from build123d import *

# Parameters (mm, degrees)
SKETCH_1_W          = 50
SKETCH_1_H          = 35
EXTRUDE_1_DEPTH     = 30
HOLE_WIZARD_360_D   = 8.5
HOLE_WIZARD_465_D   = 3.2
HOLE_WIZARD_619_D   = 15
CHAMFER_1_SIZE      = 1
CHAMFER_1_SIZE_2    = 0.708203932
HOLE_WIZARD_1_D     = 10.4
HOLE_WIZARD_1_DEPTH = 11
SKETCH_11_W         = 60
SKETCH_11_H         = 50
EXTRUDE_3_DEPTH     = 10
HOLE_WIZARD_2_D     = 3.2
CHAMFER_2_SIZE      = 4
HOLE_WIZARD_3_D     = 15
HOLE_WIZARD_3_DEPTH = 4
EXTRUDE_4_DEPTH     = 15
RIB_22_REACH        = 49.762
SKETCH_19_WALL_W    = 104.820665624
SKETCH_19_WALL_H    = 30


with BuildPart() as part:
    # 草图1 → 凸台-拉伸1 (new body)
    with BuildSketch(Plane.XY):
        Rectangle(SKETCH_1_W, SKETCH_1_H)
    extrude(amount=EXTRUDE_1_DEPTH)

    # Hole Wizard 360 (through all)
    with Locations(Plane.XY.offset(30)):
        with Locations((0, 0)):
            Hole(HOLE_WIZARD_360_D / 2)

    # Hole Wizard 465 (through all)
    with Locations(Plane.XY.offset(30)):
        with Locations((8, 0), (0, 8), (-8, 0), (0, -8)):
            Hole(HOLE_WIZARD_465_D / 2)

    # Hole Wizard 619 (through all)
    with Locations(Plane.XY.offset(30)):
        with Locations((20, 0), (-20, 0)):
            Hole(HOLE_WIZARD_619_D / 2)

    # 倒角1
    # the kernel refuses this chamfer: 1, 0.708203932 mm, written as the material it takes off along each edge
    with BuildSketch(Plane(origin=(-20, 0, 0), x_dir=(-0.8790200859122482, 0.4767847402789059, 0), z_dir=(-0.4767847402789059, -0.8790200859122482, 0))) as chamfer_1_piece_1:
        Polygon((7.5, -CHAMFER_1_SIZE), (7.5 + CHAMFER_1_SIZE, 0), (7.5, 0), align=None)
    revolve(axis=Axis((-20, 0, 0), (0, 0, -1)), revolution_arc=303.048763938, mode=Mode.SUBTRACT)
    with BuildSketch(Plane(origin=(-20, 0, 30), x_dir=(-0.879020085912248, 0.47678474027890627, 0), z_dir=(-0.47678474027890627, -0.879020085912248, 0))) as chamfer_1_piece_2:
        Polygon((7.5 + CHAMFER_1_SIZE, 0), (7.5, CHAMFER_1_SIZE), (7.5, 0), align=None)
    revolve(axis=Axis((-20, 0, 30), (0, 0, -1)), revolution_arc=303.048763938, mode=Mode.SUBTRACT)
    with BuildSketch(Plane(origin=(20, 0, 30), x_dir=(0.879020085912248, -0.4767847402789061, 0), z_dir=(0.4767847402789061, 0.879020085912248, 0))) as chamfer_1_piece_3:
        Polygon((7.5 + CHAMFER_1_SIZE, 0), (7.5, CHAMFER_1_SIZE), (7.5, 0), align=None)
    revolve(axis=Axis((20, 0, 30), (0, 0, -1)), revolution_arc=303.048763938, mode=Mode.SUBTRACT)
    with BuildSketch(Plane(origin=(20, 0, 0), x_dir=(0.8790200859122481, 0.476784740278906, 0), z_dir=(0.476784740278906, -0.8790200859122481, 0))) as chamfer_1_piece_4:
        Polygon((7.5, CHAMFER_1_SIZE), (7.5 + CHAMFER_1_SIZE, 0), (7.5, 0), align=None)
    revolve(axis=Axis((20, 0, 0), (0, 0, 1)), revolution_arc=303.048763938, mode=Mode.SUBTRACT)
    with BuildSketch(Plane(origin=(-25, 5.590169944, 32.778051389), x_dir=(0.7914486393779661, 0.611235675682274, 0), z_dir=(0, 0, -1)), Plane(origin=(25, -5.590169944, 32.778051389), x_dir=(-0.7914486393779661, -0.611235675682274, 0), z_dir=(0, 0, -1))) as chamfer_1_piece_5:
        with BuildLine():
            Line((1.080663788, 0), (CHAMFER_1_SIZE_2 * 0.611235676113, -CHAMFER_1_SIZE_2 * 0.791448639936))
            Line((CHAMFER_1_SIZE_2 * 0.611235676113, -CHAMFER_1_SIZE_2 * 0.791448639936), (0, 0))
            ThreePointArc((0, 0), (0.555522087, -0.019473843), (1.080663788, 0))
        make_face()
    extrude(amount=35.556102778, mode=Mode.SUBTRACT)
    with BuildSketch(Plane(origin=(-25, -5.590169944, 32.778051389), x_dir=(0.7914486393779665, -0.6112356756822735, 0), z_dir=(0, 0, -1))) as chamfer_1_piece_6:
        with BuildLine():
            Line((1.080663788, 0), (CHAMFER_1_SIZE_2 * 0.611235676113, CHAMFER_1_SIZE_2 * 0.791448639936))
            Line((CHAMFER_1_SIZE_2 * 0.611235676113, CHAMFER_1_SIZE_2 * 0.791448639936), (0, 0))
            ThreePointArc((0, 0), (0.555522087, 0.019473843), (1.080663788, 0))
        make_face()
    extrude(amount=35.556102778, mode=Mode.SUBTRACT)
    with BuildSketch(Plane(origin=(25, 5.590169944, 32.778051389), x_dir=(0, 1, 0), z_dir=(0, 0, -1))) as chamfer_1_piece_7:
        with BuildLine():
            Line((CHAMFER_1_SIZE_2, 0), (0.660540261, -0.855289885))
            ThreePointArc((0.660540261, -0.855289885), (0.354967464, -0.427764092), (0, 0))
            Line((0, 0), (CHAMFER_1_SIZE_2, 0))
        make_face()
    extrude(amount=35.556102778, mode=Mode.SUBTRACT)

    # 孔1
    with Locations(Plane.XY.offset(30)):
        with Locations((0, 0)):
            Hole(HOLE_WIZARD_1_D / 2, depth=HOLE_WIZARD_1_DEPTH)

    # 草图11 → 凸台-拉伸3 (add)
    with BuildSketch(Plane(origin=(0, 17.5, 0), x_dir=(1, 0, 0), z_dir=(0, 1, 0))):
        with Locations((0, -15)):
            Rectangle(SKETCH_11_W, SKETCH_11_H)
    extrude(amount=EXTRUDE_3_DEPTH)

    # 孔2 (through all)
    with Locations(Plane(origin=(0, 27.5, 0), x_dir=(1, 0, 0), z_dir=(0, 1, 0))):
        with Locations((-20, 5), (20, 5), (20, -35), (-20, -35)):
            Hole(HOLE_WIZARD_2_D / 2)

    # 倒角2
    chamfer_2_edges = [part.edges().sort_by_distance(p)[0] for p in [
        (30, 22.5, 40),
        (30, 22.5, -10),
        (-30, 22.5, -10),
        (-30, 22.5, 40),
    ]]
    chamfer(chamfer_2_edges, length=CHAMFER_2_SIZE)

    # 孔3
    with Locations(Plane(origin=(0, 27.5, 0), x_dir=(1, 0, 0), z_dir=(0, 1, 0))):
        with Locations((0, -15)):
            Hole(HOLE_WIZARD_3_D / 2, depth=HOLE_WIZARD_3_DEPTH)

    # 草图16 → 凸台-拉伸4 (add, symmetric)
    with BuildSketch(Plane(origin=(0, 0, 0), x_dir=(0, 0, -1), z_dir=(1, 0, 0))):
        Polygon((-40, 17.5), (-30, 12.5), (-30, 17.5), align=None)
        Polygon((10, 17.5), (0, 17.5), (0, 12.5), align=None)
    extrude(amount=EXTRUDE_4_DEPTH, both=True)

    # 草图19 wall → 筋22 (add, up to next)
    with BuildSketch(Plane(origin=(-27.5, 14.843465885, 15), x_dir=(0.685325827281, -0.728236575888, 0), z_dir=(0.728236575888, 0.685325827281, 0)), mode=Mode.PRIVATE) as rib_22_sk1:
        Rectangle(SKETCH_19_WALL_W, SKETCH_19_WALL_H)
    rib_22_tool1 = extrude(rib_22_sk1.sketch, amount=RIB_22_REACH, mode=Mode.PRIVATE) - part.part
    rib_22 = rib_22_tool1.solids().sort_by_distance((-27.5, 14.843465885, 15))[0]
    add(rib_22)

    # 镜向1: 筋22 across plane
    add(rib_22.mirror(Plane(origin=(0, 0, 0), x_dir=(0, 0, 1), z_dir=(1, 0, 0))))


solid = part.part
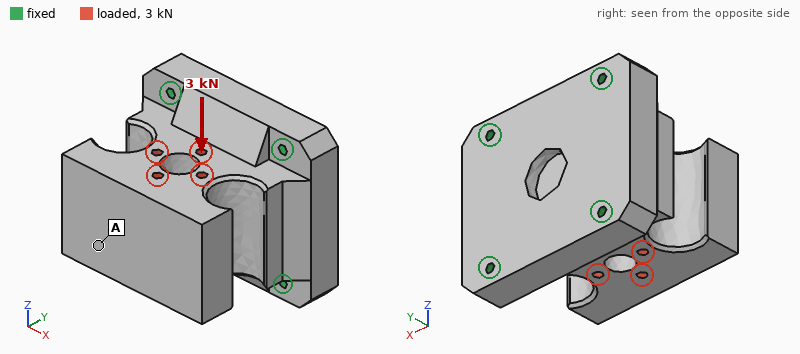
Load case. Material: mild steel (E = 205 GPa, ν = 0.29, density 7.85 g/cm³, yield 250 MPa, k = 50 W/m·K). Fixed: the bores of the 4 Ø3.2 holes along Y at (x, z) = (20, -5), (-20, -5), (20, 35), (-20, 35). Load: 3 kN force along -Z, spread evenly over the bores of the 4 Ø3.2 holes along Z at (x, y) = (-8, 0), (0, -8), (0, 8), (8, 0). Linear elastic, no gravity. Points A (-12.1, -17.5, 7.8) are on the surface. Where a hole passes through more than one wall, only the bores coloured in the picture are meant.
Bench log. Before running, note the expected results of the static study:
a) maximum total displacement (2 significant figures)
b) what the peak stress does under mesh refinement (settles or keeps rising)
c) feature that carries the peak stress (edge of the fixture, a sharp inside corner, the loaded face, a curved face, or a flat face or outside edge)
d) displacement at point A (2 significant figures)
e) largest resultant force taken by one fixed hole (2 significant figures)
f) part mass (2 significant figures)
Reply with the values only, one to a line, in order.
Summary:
4.2 µm
keeps rising
edge of the fixture
4.0 µm
1.2 kN
560 g
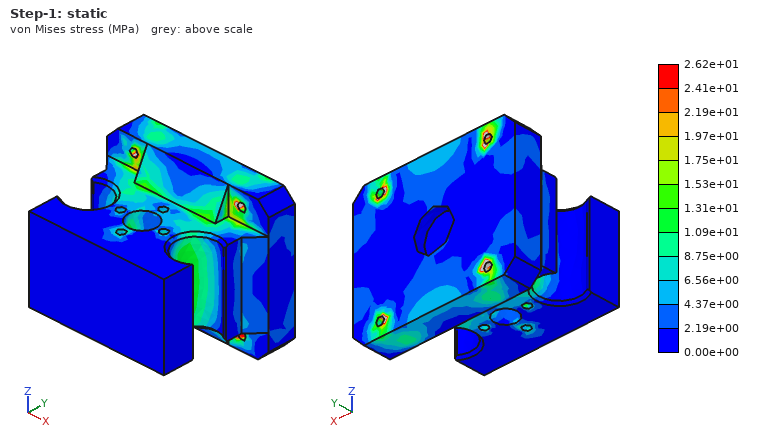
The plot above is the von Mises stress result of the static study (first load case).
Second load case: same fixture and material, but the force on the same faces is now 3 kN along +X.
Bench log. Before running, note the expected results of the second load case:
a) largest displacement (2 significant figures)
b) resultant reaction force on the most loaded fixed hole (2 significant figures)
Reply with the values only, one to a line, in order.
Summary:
4.1 µm
1.1 kN
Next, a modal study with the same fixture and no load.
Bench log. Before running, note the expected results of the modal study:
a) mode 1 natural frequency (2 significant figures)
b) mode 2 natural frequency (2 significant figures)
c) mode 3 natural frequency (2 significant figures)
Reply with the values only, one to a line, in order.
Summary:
8000 Hz
8300 Hz
11 kHz
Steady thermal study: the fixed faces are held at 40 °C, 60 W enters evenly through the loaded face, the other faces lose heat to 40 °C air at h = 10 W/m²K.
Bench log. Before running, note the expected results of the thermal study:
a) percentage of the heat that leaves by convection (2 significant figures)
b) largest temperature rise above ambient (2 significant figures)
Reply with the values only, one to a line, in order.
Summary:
5.8 %
47 K
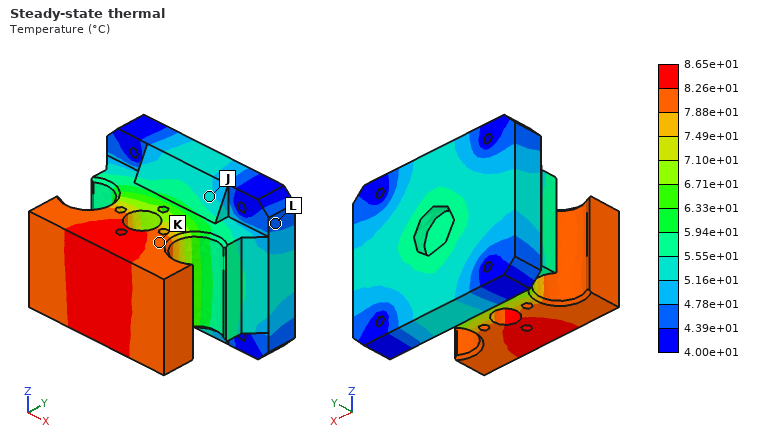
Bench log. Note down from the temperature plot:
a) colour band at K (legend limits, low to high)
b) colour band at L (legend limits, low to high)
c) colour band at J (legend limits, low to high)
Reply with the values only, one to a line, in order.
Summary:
7.88e+01 to 8.26e+01 °C
4.39e+01 to 4.78e+01 °C
5.16e+01 to 5.55e+01 °C
